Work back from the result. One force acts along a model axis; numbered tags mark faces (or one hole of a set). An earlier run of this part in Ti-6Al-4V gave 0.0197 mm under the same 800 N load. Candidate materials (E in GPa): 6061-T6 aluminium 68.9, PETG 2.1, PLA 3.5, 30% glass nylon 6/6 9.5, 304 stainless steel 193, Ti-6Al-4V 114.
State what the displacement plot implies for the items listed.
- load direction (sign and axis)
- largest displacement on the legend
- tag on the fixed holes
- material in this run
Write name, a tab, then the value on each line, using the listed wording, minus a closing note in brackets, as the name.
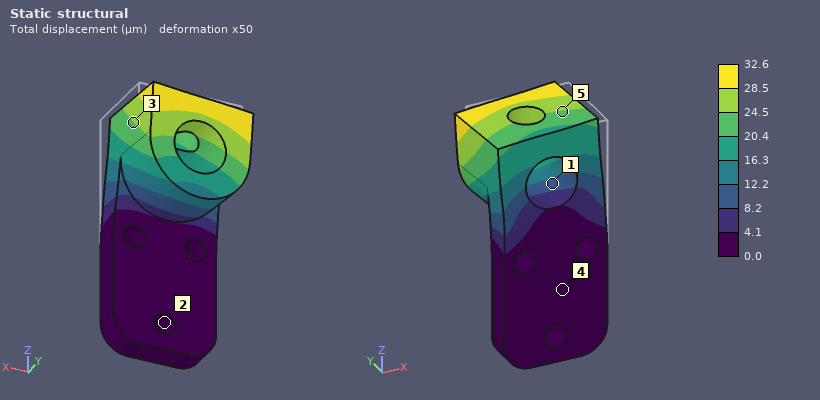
load direction	-X
largest displacement on the legend	32.6 µm
tag on the fixed holes	2
material in this run	6061-T6 aluminium
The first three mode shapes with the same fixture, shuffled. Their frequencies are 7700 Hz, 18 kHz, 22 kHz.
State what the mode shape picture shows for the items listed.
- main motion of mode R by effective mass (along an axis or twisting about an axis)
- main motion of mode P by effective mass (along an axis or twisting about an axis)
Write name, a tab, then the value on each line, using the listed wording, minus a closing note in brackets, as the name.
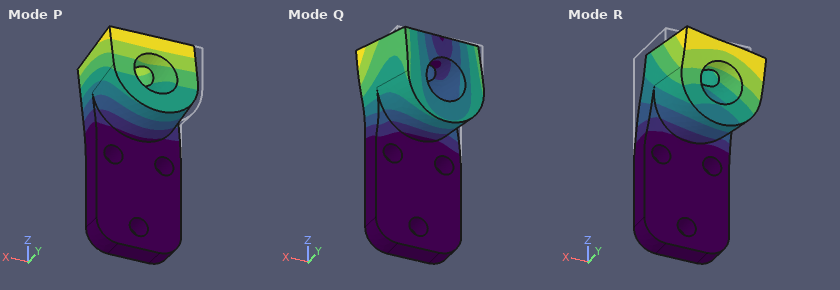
main motion of mode R by effective mass	along X
main motion of mode P by effective mass	along Y
